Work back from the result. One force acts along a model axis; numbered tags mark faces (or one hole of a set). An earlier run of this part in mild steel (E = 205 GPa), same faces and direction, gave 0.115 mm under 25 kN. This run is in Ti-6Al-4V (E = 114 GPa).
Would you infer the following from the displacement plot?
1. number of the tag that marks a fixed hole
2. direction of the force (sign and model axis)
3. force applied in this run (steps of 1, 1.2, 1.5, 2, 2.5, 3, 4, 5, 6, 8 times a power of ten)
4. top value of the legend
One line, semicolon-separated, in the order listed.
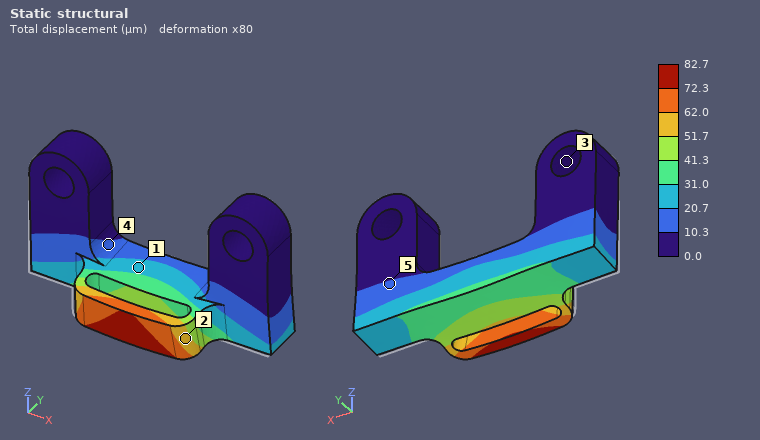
3; -Z; 10 kN; 82.7 µm
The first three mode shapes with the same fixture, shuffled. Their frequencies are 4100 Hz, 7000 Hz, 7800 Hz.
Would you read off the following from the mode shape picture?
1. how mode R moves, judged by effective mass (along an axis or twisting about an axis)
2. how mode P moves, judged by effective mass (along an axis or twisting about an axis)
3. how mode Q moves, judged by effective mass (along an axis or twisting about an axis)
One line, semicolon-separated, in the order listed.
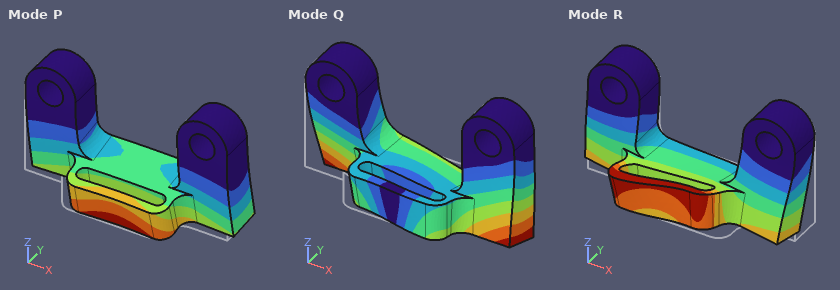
along X; along Y; along X
